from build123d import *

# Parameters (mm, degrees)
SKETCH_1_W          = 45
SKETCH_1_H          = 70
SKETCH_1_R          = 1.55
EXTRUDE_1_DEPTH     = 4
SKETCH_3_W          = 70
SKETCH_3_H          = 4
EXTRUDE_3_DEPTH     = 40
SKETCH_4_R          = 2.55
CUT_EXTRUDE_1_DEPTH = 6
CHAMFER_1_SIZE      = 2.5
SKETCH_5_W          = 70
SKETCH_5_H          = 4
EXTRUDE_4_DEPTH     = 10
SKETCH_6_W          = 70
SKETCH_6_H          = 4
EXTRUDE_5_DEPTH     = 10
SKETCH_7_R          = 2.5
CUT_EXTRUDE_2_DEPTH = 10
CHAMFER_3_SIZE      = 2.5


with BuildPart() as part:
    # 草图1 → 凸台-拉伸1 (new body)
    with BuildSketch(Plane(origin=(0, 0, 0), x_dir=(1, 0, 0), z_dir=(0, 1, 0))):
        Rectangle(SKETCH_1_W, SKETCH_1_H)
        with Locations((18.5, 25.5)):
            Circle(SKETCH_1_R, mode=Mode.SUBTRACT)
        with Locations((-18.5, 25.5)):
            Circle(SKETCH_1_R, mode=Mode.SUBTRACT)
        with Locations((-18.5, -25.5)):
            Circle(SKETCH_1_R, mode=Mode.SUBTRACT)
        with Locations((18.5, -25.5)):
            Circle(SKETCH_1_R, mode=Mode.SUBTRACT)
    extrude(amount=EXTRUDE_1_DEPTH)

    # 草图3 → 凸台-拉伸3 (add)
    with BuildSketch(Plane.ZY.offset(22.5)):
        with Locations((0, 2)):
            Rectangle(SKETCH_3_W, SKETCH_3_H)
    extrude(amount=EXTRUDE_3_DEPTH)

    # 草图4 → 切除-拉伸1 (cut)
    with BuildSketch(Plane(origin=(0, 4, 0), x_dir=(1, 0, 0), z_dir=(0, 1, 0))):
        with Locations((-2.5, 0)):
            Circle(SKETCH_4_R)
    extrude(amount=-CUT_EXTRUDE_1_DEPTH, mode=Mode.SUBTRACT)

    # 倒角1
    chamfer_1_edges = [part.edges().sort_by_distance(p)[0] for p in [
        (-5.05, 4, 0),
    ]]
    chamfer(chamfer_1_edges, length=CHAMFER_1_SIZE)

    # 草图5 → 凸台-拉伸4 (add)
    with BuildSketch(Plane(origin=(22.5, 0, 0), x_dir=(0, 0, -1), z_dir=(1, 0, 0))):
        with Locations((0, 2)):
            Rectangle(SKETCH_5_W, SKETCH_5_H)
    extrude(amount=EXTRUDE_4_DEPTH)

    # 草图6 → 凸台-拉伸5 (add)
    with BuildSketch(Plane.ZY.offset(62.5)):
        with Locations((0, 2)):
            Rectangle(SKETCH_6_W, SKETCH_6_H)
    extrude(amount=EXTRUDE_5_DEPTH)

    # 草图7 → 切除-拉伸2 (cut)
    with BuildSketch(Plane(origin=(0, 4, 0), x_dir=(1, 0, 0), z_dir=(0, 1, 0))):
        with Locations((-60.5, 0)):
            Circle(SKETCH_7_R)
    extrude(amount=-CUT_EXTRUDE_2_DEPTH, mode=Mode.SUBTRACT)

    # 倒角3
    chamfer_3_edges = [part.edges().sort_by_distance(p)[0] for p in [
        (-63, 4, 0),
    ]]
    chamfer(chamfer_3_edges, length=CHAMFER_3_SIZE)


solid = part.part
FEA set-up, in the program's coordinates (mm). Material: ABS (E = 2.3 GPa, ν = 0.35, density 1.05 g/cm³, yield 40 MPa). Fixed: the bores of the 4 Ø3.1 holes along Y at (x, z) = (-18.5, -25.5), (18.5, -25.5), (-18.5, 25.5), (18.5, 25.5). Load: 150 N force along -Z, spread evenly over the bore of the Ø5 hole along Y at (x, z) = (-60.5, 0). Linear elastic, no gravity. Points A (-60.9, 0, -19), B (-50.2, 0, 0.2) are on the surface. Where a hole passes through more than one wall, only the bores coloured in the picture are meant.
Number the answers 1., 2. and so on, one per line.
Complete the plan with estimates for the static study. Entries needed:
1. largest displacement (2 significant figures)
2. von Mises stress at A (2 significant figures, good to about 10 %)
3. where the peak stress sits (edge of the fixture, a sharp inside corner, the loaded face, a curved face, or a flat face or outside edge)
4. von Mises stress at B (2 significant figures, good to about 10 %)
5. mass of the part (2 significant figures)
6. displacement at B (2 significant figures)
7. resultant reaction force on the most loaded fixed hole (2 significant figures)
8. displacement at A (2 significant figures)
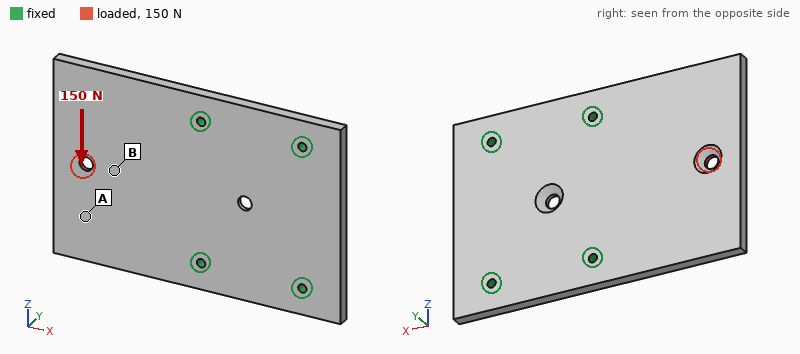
1. 0.16 mm
2. 1.1 MPa
3. the loaded face
4. 2.5 MPa
5. 30 g
6. 0.046 mm
7. 130 N
8. 0.093 mm
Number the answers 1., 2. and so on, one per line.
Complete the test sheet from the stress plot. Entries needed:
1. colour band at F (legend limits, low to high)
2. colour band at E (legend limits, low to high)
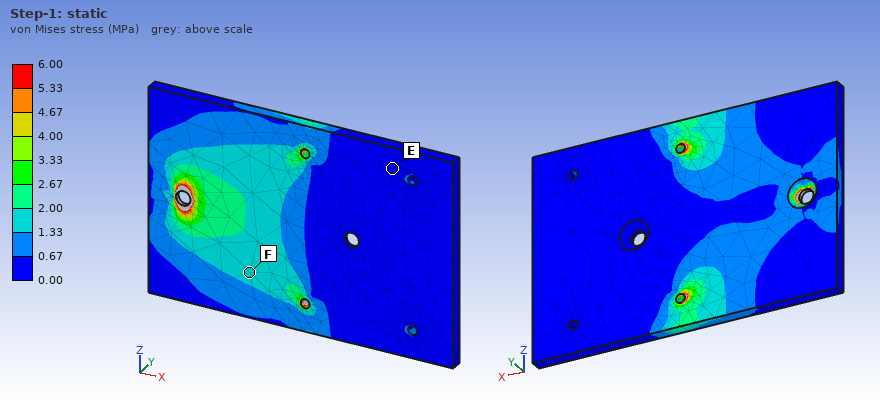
1. 1.33 to 2.00 MPa
2. 0.00 to 0.67 MPa
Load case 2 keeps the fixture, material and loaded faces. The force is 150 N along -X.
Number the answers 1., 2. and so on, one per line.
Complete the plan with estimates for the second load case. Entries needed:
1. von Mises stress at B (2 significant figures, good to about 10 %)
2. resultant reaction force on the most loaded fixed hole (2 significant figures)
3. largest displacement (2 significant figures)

1. 2.8 MPa
2. 58 N
3. 0.36 mm
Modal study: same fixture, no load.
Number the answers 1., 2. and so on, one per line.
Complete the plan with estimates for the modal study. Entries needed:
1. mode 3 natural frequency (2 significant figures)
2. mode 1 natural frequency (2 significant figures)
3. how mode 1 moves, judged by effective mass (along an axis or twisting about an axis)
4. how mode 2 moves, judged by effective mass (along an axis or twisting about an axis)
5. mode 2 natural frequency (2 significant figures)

1. 1500 Hz
2. 300 Hz
3. along Y
4. twisting about X
5. 640 Hz
